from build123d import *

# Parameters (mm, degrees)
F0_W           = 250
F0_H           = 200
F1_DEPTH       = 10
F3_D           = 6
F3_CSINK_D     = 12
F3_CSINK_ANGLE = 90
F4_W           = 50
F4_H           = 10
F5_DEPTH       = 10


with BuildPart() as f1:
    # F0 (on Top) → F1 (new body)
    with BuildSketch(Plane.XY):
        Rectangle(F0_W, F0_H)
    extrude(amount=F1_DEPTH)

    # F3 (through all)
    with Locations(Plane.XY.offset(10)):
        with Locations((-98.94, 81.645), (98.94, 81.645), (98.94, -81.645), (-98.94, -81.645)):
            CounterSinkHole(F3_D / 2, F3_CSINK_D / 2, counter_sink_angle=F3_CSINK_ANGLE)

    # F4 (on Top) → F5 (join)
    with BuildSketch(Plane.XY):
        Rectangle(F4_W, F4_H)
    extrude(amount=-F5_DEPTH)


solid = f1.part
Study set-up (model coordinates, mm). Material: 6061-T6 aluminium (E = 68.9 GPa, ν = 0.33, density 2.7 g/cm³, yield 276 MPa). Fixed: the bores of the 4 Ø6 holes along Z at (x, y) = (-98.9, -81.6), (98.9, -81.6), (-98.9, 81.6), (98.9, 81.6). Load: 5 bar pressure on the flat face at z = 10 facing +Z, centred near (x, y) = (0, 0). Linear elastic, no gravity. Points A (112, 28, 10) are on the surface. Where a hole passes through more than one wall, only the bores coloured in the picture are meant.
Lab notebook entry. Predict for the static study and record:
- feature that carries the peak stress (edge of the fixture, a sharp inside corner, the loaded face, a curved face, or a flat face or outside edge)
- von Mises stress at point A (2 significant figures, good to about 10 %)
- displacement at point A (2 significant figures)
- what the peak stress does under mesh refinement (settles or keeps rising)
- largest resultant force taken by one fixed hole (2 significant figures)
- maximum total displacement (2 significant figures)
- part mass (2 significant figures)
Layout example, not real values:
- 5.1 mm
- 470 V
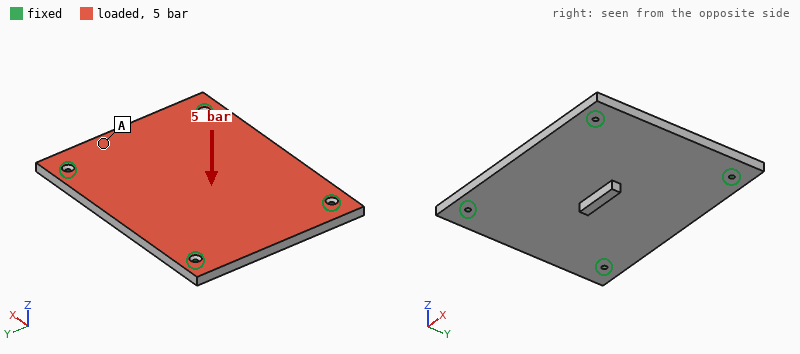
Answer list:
- edge of the fixture
- 44 MPa
- 0.23 mm
- keeps rising
- 7.0 kN
- 0.84 mm
- 1.4 kg
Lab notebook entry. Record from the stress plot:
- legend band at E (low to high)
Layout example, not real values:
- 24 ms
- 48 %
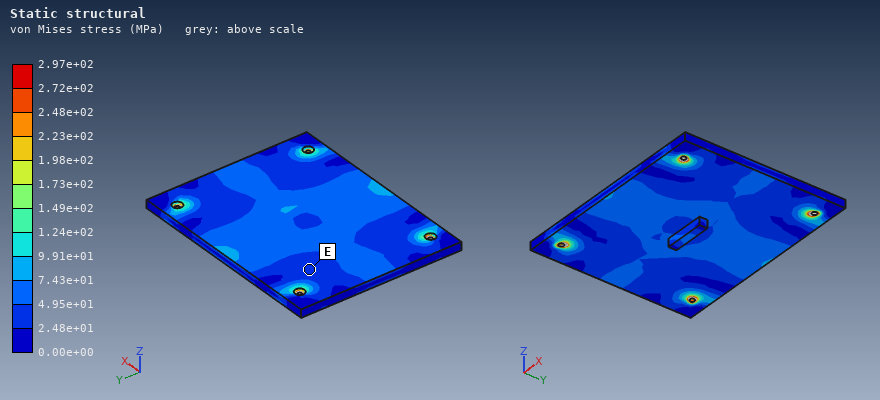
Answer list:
- 2.48e+01 to 4.95e+01 MPa
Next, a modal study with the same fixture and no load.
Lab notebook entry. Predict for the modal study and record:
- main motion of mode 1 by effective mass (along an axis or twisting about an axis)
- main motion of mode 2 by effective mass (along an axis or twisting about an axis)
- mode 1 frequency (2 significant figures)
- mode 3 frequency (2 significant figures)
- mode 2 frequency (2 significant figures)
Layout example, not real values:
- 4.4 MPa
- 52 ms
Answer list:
- along Z
- twisting about X
- 860 Hz
- 1600 Hz
- 1400 Hz
